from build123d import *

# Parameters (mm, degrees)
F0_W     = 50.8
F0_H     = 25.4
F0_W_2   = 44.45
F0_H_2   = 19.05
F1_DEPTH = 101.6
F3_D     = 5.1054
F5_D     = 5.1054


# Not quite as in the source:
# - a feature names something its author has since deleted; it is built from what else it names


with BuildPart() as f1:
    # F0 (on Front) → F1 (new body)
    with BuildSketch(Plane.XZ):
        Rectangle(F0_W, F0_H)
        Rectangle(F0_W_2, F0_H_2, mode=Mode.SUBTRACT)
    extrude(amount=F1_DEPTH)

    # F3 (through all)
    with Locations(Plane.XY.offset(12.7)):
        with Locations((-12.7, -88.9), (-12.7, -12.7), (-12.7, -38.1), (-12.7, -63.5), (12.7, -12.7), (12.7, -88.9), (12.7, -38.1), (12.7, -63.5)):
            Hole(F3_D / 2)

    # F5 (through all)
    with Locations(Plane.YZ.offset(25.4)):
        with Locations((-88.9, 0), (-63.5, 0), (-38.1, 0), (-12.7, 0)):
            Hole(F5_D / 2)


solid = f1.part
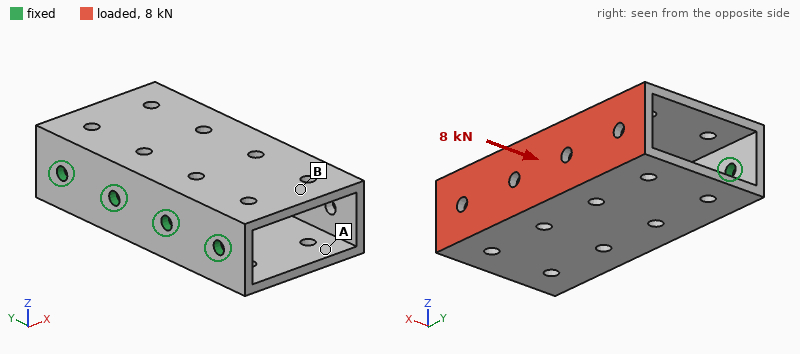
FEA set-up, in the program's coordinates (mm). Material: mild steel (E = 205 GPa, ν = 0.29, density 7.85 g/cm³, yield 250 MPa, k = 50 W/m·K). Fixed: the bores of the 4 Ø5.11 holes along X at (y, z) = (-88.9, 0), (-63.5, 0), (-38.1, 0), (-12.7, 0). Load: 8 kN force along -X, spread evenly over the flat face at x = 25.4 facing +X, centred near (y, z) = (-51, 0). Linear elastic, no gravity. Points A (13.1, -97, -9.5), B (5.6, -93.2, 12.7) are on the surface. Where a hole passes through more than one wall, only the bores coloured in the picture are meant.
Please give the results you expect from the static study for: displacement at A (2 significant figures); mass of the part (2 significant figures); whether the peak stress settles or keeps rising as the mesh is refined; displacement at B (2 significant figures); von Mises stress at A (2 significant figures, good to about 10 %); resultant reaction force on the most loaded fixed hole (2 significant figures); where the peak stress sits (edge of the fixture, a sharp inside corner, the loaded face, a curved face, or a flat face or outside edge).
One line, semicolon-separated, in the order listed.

31 µm; 340 g; keeps rising; 33 µm; 41 MPa; 2.0 kN; edge of the fixture
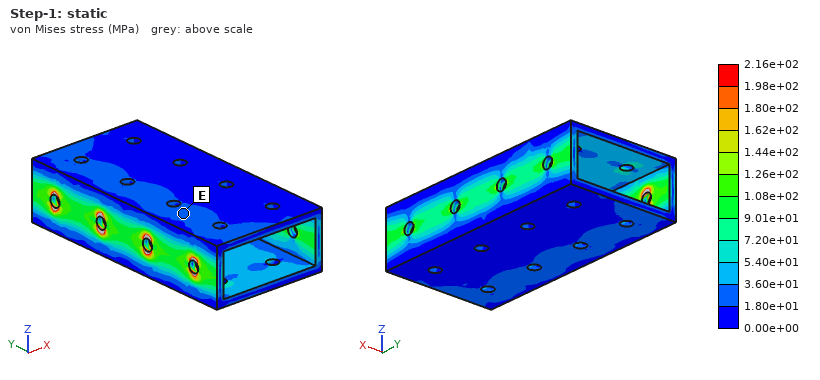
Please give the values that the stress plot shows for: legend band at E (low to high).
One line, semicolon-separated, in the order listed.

1.80e+01 to 3.60e+01 MPa
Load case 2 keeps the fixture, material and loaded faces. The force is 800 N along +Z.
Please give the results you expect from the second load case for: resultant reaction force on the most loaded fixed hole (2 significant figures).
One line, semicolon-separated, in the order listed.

230 N
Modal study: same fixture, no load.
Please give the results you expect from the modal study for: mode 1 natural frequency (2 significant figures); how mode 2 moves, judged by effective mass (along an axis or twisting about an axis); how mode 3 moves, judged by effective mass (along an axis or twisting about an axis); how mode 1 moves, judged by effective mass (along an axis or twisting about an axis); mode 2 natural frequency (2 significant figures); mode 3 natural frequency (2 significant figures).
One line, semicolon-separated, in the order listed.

900 Hz; twisting about X; along Y; along Z; 2700 Hz; 3600 Hz
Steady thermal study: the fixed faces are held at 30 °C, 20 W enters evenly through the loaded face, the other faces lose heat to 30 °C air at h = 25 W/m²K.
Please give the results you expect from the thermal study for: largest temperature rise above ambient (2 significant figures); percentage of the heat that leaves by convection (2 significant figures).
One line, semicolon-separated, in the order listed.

29 K; 46 %
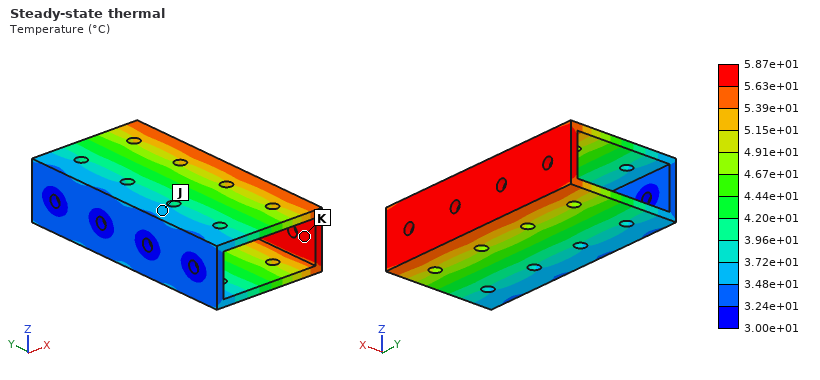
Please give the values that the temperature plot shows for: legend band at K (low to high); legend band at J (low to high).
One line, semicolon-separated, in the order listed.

5.63e+01 to 5.87e+01 °C; 3.48e+01 to 3.72e+01 °C
